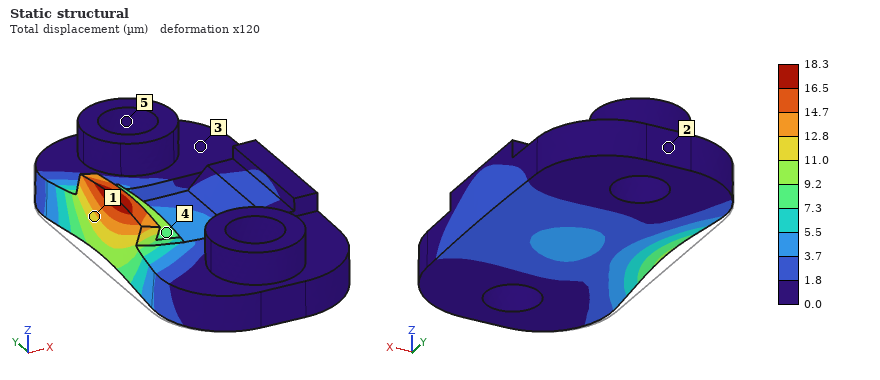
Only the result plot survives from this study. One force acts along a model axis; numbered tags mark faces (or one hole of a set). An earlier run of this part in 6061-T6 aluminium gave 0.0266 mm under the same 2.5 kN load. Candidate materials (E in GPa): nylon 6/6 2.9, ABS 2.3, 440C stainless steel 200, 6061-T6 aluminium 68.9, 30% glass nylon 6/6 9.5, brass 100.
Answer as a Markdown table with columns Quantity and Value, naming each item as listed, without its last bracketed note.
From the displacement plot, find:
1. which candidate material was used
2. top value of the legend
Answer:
| Quantity | Value |
|---|---|
| which candidate material was used | brass |
| top value of the legend | 18.3 µm |
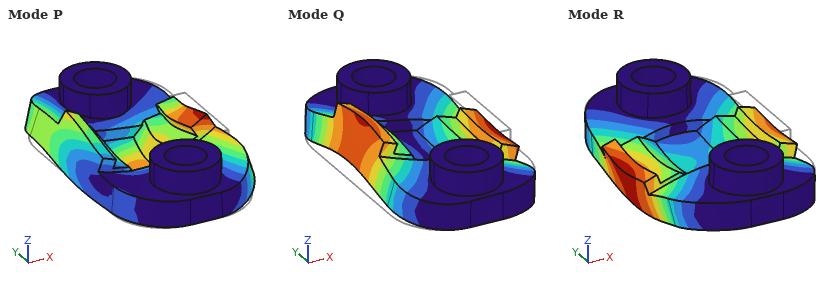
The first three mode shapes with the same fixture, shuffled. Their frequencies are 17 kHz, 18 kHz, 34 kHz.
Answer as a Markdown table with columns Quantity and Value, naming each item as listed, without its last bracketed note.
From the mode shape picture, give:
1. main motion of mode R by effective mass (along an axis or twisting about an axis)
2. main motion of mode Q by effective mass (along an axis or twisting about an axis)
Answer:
| Quantity | Value |
|---|---|
| main motion of mode R by effective mass | along Z |
| main motion of mode Q by effective mass | twisting about Y |
